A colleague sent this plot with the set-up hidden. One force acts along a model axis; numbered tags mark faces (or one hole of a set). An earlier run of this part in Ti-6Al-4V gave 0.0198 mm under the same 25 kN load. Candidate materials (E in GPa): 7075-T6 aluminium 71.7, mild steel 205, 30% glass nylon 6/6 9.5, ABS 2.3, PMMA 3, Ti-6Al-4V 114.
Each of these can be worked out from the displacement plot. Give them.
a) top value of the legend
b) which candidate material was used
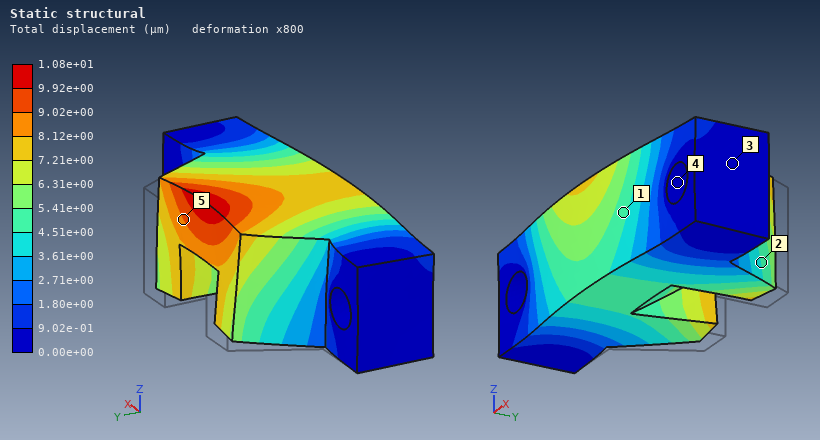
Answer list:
1.08e+01 µm
mild steel
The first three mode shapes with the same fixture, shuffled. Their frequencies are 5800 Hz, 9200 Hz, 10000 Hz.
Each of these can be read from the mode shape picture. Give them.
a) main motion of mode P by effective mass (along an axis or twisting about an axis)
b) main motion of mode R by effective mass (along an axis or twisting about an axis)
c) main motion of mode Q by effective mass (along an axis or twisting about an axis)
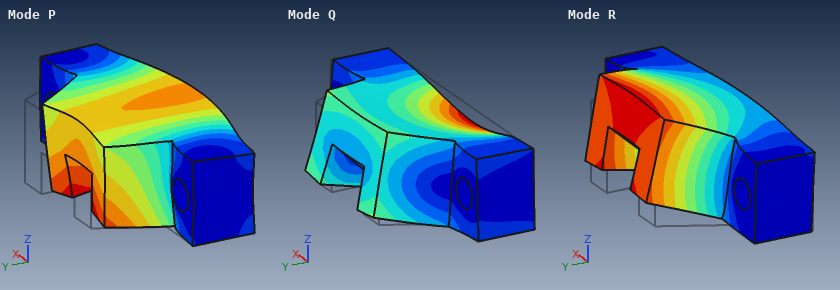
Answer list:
along Y
along Z
along Z
